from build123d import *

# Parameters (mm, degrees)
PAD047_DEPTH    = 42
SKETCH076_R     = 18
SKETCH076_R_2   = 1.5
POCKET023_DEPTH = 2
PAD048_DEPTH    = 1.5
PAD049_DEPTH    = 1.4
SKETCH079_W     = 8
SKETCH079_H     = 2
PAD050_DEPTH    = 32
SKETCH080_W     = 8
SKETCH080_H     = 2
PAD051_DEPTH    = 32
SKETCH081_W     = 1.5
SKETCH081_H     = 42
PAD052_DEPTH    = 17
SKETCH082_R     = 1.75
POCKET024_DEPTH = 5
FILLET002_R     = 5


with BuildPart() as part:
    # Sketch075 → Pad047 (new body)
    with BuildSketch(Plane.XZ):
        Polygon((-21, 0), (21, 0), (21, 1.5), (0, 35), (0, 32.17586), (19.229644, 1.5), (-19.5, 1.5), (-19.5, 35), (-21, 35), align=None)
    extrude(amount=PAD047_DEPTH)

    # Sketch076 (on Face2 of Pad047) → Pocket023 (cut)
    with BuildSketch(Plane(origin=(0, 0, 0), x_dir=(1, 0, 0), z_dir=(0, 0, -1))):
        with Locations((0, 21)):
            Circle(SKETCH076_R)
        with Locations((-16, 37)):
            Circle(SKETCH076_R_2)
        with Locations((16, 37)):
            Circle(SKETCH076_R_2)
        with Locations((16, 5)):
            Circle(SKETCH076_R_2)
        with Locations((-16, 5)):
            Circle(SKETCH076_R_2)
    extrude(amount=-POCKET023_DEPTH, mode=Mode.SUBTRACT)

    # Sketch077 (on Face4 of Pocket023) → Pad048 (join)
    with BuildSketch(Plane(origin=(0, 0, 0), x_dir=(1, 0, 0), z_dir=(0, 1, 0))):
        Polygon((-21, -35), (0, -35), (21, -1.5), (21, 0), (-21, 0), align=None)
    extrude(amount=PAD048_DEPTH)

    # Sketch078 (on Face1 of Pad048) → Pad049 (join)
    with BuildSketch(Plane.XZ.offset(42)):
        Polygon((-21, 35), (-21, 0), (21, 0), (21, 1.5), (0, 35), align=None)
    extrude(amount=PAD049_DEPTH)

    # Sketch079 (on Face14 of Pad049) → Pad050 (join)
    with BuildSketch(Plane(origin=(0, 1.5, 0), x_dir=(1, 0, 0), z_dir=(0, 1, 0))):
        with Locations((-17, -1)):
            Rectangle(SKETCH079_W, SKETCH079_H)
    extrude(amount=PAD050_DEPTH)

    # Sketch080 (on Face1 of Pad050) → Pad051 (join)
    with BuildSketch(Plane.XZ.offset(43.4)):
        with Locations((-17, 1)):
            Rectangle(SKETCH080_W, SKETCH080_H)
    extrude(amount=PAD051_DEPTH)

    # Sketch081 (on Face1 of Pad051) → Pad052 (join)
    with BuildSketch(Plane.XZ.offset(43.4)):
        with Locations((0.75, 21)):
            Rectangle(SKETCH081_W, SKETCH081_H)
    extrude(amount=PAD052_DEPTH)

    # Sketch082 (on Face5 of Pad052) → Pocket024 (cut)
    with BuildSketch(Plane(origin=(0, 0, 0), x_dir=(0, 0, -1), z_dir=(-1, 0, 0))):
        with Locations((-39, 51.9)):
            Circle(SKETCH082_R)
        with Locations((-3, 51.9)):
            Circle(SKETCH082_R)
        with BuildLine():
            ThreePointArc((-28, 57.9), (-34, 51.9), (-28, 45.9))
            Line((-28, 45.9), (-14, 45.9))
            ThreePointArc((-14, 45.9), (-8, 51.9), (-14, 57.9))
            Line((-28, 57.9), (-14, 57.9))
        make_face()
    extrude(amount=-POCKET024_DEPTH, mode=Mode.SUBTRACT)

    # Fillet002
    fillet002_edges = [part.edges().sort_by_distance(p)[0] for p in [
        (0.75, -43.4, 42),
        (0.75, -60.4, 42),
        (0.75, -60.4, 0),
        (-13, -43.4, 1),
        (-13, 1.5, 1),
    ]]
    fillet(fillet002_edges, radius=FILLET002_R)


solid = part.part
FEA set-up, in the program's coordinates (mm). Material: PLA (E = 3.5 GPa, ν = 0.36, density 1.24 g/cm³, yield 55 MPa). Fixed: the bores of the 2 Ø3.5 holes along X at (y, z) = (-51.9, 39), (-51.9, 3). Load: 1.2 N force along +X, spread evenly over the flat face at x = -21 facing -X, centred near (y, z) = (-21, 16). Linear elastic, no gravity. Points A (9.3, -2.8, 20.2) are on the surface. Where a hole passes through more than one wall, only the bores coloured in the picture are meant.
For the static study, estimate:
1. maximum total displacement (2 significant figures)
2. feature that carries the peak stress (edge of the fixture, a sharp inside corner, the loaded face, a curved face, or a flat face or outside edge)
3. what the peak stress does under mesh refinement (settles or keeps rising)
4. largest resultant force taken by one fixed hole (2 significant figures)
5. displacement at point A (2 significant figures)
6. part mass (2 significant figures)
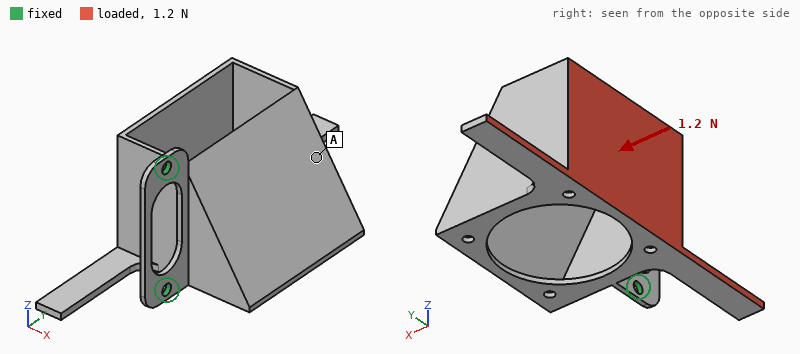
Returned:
1.4 mm
edge of the fixture
keeps rising
1.0 N
0.74 mm
13 g
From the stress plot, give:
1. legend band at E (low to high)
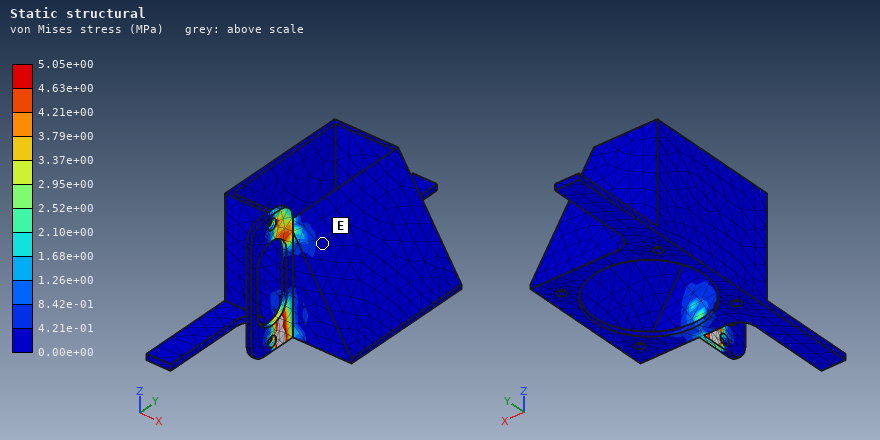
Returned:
0.00e+00 to 4.21e-01 MPa
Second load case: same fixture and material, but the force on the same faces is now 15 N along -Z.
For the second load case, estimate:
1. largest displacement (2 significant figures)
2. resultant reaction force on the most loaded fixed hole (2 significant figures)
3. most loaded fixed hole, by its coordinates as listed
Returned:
1.1 mm
18 N
(-51.9, 39)
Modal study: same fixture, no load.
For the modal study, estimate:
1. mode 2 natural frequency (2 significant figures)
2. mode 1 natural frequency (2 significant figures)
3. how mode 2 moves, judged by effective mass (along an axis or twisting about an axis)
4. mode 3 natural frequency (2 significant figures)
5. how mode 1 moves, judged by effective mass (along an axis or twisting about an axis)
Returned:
280 Hz
55 Hz
along Z
470 Hz
along X
